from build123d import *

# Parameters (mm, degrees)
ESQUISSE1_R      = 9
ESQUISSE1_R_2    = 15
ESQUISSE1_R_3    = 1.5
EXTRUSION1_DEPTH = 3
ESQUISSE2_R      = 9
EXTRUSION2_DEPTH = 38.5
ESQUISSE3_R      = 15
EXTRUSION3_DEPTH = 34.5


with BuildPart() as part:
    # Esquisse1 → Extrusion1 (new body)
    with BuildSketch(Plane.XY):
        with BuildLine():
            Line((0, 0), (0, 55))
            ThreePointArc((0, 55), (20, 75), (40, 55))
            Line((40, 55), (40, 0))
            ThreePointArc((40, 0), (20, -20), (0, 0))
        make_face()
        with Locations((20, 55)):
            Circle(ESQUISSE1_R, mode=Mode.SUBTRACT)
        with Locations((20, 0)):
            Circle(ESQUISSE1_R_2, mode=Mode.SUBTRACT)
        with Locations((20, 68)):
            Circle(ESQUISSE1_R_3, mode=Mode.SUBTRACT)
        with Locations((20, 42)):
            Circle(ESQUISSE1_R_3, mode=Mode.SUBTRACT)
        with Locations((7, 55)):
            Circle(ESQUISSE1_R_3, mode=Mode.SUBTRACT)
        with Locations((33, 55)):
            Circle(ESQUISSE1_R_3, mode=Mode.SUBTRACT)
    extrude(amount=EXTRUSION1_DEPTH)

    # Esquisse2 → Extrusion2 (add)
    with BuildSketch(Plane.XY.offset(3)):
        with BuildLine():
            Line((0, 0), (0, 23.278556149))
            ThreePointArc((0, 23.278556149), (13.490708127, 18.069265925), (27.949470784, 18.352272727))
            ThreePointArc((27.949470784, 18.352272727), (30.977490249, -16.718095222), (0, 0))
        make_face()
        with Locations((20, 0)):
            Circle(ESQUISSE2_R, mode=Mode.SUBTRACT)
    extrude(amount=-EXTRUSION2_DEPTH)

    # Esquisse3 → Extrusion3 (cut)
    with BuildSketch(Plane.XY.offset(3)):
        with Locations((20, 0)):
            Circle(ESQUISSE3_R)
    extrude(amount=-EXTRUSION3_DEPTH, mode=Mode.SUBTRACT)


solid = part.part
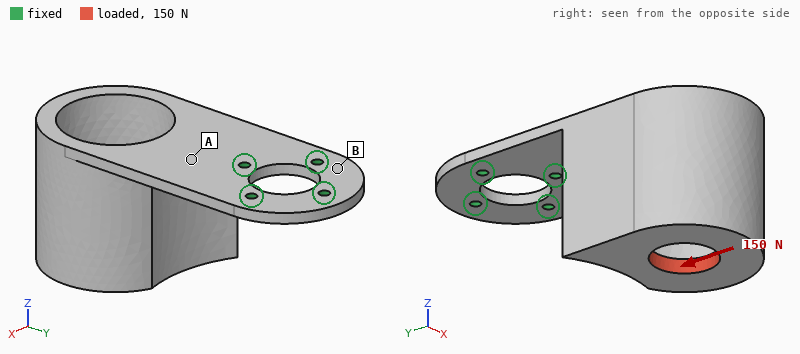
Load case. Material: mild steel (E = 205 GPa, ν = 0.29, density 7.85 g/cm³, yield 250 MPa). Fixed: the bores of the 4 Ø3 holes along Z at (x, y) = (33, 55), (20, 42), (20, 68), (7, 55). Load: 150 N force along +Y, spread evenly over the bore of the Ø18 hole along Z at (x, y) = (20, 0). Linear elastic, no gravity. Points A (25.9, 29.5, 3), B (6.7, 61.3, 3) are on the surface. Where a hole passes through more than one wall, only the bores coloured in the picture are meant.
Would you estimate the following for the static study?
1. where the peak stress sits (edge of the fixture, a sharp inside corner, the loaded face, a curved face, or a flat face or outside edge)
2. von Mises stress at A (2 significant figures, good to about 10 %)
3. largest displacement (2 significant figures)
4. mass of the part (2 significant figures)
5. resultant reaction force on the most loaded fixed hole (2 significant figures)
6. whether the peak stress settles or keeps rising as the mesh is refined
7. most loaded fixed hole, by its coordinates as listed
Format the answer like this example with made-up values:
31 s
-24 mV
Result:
edge of the fixture
75 MPa
0.46 mm
240 g
240 N
keeps rising
(20, 42)
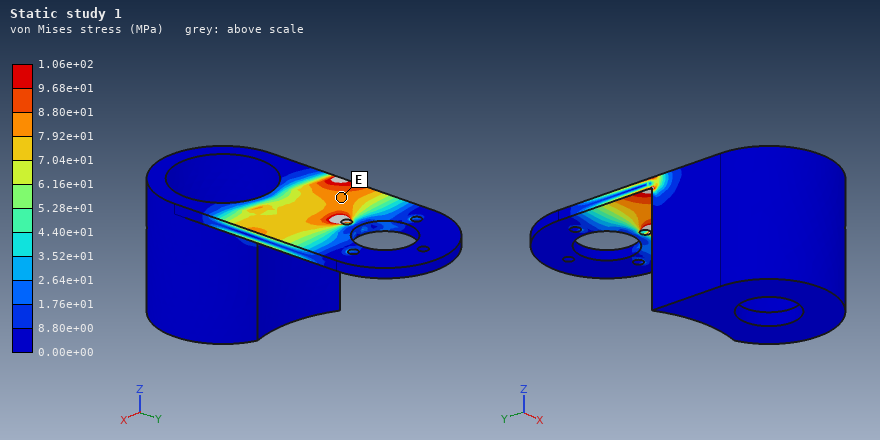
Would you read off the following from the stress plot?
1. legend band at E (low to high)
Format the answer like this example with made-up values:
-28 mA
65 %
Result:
7.92e+01 to 8.80e+01 MPa
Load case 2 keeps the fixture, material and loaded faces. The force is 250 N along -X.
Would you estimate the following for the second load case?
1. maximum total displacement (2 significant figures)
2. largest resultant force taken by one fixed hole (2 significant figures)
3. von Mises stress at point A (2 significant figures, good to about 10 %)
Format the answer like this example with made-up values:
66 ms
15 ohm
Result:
0.26 mm
350 N
79 MPa
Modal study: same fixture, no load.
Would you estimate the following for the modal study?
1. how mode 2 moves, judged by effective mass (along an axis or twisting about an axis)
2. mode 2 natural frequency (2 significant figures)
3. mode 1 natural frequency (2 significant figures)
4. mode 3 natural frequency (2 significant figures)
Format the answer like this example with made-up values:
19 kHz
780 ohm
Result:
along X
520 Hz
240 Hz
1600 Hz
